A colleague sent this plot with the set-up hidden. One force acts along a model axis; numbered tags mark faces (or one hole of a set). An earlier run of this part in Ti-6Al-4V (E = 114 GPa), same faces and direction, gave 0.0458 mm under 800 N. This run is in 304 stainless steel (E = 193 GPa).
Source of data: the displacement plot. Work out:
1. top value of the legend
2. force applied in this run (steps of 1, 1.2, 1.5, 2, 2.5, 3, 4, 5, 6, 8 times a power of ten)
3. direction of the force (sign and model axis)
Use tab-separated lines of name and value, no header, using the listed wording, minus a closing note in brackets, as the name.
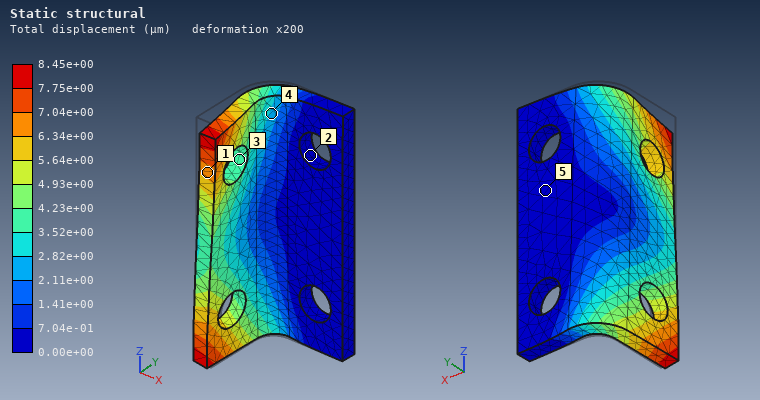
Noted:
top value of the legend	8.45e+00 µm
force applied in this run	250 N
direction of the force	-Z
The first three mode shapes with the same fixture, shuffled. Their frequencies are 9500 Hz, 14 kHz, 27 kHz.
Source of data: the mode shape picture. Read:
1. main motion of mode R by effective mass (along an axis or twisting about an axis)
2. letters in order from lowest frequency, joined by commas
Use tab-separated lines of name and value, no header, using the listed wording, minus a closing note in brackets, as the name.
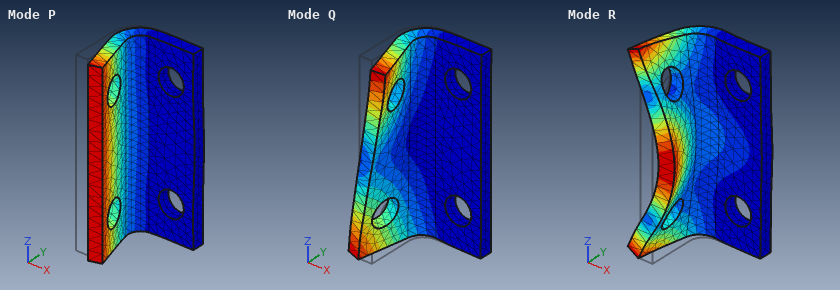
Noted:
main motion of mode R by effective mass	along Y
letters in order from lowest frequency, joined by commas	P, Q, R
